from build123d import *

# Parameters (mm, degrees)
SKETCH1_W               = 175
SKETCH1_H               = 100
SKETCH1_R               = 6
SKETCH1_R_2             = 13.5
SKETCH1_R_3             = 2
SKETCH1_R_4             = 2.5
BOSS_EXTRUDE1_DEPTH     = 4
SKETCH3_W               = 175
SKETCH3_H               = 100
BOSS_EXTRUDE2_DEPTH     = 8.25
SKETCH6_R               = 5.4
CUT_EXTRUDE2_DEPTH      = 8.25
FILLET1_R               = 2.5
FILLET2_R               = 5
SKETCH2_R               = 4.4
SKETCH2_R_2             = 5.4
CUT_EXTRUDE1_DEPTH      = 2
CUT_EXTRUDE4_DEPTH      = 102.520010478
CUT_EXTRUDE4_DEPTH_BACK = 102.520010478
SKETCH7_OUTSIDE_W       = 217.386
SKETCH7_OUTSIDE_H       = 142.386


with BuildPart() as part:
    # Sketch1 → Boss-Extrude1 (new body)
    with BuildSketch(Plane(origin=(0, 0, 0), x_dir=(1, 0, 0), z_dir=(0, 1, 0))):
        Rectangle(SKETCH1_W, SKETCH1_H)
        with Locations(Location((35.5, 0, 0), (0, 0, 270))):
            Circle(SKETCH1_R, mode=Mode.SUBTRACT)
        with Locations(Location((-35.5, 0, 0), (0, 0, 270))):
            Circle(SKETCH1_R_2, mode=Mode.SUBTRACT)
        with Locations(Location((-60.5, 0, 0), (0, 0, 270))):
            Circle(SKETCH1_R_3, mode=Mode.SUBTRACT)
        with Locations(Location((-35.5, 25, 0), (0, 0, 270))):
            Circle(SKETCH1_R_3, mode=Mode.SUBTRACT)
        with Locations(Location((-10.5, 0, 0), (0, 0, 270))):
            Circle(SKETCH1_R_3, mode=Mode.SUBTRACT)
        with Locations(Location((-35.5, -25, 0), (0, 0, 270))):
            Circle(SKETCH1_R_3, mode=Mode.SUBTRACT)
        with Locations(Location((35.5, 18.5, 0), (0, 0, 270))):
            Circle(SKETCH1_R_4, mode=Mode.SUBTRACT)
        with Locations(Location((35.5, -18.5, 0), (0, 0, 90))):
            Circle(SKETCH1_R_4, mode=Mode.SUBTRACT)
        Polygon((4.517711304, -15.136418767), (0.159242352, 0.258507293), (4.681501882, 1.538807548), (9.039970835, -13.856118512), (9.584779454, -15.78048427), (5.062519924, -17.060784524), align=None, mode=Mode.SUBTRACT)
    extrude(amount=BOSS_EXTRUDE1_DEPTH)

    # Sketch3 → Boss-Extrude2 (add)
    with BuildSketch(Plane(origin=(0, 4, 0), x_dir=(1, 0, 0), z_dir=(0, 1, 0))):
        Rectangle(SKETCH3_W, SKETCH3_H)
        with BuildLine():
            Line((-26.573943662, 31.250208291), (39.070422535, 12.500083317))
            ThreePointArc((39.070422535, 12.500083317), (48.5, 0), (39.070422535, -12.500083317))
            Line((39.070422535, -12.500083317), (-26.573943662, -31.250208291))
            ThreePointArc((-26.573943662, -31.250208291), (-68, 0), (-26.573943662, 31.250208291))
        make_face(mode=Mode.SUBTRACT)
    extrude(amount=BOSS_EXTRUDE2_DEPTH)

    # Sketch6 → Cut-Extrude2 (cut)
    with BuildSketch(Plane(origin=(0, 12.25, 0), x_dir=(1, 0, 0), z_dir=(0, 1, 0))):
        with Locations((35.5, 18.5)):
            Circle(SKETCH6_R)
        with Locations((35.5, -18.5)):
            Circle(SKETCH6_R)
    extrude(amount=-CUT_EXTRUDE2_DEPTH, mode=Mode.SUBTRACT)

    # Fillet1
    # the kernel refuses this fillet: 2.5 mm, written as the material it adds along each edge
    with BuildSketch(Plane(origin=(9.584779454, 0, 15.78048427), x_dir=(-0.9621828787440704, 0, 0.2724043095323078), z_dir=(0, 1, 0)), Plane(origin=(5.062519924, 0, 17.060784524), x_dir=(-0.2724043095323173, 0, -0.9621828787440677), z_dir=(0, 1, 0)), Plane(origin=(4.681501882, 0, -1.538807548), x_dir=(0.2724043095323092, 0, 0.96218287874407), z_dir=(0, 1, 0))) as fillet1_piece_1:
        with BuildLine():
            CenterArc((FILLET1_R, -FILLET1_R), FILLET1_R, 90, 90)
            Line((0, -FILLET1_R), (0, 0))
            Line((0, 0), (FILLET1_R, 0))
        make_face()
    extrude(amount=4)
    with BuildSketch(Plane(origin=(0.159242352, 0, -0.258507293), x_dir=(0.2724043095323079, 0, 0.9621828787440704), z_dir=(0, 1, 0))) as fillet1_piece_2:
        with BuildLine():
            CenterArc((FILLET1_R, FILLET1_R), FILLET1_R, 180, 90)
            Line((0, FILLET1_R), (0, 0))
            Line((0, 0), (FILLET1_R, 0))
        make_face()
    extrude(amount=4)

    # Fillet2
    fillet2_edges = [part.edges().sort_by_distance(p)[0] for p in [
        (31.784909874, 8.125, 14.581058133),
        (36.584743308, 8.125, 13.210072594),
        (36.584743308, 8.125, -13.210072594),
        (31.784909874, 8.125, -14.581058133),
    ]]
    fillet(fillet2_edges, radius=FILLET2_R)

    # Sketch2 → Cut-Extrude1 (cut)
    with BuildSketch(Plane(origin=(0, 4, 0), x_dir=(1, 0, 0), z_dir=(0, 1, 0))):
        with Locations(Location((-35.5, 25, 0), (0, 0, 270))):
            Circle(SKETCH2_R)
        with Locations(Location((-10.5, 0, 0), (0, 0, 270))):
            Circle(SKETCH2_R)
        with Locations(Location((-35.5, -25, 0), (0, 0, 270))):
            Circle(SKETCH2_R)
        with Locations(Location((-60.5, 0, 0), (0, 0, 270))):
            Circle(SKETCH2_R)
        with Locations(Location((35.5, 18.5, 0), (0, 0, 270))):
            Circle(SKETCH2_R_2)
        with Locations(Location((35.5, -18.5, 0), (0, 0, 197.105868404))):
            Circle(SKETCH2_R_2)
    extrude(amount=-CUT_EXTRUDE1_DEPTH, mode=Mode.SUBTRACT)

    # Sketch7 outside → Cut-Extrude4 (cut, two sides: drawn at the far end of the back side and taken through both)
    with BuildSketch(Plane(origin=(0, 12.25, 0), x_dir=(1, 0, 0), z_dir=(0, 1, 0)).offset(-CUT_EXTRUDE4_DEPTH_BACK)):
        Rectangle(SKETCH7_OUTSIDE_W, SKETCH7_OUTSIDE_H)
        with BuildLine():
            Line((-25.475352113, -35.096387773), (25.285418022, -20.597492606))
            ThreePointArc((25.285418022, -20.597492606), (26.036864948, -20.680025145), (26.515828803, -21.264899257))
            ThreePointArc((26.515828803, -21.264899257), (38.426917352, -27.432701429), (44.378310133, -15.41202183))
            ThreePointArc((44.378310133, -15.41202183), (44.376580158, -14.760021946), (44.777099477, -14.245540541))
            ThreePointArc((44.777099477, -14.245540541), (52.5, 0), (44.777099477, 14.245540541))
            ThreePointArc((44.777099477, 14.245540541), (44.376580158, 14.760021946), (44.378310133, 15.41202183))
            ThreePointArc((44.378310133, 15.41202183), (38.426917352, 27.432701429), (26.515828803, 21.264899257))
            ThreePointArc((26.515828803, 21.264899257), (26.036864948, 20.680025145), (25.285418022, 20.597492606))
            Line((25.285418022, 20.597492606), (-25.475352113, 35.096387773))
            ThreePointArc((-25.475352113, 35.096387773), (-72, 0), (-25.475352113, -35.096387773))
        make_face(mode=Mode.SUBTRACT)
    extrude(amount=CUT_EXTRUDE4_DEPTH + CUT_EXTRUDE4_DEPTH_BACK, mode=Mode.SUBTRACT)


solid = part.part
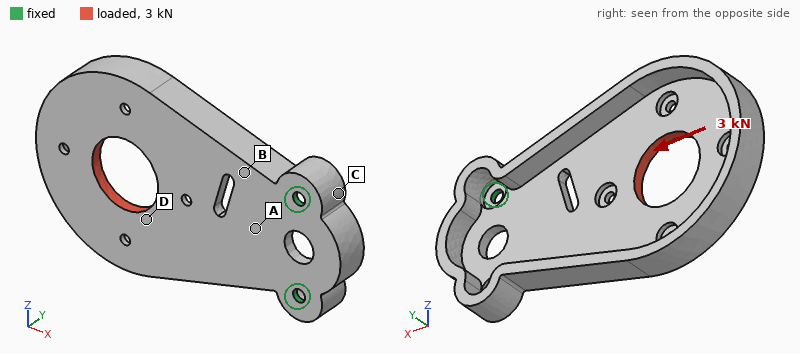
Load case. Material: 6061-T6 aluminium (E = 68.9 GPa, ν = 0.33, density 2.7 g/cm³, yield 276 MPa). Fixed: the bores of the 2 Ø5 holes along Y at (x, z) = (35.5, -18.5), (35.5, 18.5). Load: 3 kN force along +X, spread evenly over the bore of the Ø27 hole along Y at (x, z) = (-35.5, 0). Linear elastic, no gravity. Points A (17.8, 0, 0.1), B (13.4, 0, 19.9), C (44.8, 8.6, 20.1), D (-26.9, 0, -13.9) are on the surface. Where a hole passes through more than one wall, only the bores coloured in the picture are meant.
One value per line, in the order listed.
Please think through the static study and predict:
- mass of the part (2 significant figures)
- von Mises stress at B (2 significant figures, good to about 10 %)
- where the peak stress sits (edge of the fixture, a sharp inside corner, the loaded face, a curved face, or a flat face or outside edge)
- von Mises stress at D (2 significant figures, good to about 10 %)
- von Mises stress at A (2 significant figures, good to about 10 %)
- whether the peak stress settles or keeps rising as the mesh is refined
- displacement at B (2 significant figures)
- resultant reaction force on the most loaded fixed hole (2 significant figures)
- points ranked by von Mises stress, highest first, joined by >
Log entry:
92 g
33 MPa
edge of the fixture
23 MPa
12 MPa
keeps rising
29 µm
1.5 kN
B > D > A > C
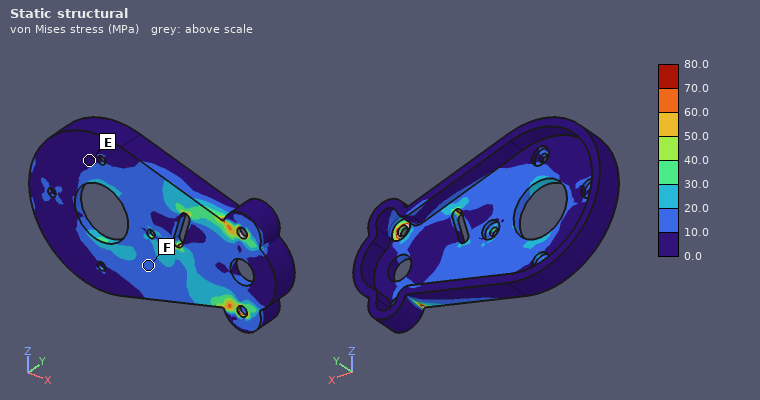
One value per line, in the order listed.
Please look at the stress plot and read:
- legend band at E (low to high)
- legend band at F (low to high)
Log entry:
0.0 to 10.0 MPa
10.0 to 20.0 MPa
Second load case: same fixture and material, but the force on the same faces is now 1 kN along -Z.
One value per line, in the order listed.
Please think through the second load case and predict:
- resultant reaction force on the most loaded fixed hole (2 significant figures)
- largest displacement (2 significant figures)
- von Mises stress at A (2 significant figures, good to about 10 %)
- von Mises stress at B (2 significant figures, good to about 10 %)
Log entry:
1.9 kN
0.14 mm
22 MPa
33 MPa
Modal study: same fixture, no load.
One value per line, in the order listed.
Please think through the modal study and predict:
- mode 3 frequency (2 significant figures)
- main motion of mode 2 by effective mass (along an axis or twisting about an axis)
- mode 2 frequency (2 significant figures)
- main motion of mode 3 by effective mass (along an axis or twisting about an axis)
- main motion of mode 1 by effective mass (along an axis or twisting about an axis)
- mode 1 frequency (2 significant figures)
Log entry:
2000 Hz
twisting about X
920 Hz
along Z
along Y
320 Hz
